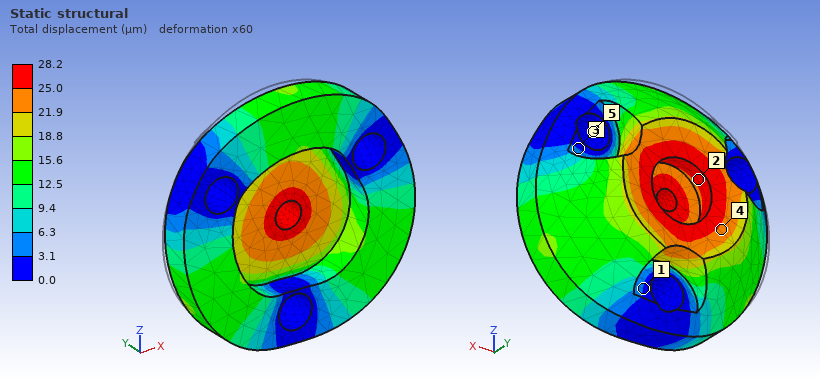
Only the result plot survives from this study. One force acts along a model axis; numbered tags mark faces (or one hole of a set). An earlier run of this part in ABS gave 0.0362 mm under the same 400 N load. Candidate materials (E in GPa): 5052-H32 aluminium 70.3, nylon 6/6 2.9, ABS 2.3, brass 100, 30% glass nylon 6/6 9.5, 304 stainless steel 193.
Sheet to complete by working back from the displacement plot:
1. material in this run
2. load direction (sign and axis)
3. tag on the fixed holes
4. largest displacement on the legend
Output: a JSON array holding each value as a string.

["nylon 6/6", "-Y", "5", "28.2 µm"]
